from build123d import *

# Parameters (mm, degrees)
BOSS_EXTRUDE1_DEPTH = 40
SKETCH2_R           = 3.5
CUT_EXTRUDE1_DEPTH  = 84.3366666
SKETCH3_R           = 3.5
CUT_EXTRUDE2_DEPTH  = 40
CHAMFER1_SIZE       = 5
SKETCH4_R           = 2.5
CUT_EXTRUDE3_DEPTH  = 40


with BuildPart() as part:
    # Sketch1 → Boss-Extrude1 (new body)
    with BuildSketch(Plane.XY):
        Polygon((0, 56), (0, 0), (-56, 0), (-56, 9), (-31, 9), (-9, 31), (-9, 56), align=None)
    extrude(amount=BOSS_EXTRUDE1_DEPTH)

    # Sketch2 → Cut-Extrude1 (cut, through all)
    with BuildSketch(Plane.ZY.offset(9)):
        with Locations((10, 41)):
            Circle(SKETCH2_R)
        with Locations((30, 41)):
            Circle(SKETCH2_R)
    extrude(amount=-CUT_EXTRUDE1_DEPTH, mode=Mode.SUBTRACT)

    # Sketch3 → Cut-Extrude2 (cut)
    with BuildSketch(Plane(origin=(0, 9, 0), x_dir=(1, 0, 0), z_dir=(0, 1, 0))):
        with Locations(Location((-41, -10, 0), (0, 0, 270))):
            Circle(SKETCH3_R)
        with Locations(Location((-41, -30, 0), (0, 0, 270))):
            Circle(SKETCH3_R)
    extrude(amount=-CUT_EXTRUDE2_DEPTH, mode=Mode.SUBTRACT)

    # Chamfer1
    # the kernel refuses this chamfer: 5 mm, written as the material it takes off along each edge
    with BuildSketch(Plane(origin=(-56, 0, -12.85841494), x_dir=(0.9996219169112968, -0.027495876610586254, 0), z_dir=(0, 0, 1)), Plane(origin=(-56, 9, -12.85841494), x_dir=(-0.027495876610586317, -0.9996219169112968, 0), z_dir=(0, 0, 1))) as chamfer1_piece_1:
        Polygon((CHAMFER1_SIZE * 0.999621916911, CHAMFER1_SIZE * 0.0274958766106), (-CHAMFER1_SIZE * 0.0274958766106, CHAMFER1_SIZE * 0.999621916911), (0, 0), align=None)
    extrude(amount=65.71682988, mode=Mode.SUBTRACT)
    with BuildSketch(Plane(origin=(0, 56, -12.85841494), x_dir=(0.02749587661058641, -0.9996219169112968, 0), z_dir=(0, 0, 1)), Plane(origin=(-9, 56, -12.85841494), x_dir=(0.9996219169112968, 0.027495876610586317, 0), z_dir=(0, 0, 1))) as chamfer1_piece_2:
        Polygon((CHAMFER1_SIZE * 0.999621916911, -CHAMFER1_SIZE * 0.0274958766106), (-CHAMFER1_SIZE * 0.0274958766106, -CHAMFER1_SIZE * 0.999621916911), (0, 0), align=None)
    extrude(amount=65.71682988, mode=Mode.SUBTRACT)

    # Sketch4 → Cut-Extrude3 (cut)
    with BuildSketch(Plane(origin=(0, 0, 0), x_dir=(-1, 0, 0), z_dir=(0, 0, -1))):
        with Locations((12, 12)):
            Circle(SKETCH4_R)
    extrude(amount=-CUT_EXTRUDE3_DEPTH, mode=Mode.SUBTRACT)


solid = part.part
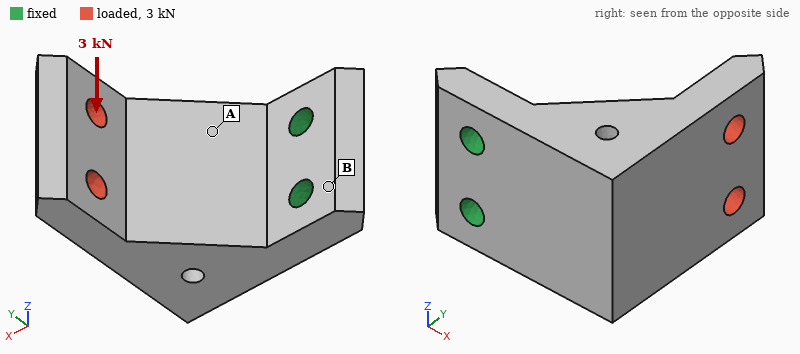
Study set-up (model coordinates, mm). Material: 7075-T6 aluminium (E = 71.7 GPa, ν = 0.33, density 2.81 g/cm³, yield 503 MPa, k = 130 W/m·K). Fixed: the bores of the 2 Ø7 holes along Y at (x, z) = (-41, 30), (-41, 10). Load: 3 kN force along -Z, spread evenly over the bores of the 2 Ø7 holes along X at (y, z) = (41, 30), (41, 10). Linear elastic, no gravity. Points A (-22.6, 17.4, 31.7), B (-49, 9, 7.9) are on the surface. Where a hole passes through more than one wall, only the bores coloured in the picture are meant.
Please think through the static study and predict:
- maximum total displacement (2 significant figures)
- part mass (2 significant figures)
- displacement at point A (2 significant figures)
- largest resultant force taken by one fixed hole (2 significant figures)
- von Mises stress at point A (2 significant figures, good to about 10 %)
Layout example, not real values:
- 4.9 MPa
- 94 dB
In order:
- 0.18 mm
- 120 g
- 0.050 mm
- 6.0 kN
- 44 MPa
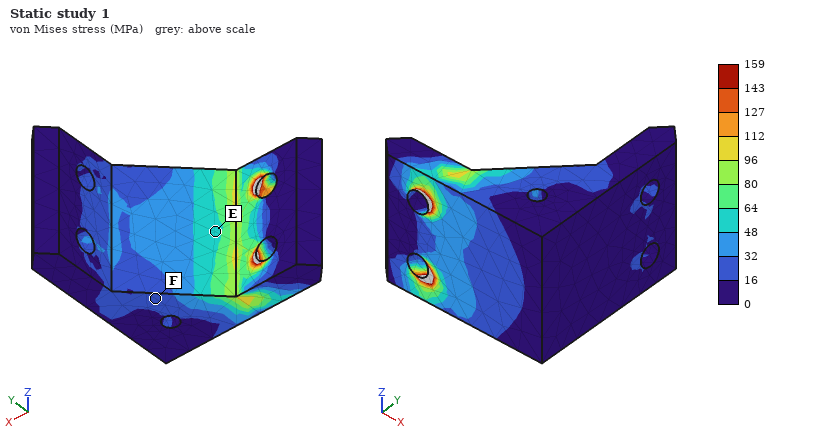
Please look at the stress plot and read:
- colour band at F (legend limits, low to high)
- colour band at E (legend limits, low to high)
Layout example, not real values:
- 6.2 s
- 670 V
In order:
- 16 to 32 MPa
- 48 to 64 MPa
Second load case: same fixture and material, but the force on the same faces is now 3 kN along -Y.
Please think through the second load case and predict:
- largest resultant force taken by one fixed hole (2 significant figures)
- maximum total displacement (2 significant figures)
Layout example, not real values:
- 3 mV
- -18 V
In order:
- 1.5 kN
- 0.41 mm
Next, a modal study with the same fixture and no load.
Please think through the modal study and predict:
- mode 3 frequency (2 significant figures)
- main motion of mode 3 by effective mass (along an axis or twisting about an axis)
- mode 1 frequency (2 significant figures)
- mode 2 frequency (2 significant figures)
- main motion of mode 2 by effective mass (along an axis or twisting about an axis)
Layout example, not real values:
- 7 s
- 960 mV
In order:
- 7800 Hz
- along Z
- 1800 Hz
- 4000 Hz
- along Z
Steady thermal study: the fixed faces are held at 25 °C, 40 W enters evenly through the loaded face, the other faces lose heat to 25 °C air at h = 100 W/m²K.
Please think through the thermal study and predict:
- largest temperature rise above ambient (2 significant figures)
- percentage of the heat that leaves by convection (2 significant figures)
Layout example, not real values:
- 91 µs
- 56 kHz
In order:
- 31 K
- 34 %
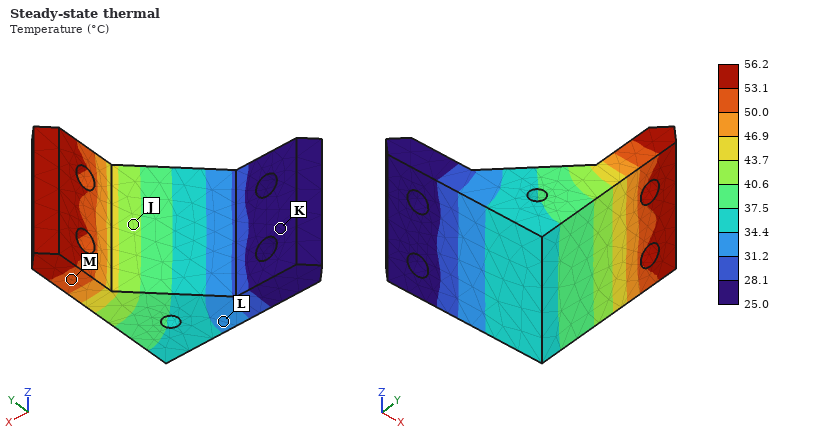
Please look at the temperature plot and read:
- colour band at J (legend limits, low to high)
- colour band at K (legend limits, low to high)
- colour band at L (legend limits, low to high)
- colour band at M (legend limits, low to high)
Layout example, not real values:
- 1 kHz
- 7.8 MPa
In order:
- 40.6 to 43.7 °C
- 25.0 to 28.1 °C
- 31.2 to 34.4 °C
- 50.0 to 53.1 °C
